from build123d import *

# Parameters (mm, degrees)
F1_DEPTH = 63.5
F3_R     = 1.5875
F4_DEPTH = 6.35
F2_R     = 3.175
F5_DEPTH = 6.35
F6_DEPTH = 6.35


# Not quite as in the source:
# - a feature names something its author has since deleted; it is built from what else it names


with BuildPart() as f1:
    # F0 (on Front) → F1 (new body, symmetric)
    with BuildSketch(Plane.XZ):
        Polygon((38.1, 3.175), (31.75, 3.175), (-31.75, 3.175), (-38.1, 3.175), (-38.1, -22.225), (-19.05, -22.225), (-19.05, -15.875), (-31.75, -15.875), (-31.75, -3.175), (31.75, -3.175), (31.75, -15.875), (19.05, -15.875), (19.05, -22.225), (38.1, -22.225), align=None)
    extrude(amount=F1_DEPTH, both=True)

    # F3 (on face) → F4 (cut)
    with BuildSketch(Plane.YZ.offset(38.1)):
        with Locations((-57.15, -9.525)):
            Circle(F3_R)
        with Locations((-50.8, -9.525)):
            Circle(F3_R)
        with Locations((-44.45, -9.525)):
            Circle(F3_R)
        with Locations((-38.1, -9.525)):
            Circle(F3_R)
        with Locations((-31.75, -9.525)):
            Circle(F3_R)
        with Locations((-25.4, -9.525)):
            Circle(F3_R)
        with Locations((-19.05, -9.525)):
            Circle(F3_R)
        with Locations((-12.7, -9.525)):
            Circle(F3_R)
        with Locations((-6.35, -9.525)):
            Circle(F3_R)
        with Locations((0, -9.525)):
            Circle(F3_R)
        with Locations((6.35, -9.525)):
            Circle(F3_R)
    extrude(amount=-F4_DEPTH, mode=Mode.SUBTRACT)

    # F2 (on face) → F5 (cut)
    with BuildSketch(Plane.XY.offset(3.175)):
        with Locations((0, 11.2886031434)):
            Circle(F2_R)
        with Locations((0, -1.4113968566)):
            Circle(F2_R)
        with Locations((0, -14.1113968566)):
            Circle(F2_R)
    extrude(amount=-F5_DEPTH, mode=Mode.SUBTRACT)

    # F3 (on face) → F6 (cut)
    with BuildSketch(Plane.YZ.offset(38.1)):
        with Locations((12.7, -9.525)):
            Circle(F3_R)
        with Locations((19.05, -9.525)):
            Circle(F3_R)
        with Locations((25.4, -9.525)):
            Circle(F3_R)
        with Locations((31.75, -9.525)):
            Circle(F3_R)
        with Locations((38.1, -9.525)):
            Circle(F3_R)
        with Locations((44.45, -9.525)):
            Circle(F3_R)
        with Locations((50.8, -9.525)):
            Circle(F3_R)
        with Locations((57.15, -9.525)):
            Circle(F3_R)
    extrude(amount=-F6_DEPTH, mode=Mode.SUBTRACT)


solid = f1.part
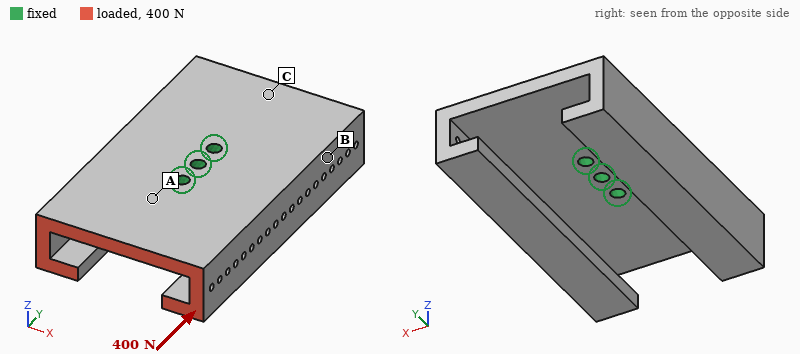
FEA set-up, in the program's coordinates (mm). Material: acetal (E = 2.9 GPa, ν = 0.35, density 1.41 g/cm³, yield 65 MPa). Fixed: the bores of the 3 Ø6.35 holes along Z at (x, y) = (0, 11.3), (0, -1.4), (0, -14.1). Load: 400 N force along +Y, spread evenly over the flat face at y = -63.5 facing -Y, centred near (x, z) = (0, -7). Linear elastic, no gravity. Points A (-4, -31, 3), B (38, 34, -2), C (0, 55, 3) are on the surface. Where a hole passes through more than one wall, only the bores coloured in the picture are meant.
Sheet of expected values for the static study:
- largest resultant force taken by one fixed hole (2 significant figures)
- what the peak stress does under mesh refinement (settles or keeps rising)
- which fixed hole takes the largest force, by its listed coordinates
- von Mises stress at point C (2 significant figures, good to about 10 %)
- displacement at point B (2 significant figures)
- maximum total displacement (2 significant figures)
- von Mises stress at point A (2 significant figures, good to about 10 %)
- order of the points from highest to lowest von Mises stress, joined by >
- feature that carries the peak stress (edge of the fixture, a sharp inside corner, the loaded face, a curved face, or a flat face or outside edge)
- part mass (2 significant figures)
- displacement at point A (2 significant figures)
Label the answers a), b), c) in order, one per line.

a) 200 N
b) keeps rising
c) (0, -14.1)
d) 0.86 MPa
e) 0.100 mm
f) 0.20 mm
g) 1.6 MPa
h) A > C > B
i) edge of the fixture
j) 160 g
k) 0.034 mm
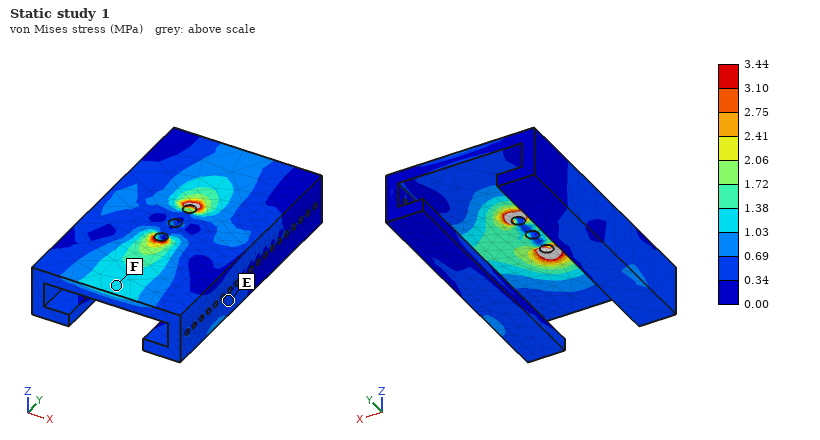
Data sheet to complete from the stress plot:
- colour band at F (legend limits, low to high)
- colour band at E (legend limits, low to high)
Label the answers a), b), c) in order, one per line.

a) 1.03 to 1.38 MPa
b) 0.34 to 0.69 MPa
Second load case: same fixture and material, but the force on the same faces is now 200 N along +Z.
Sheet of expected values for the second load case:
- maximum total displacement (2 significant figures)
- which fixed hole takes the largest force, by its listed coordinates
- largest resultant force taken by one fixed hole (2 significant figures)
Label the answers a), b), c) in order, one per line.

a) 0.93 mm
b) (0, -14.1)
c) 400 N
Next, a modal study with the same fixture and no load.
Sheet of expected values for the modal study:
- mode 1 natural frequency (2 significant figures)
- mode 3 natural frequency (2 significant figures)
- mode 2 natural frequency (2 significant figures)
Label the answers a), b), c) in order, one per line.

a) 370 Hz
b) 430 Hz
c) 370 Hz
